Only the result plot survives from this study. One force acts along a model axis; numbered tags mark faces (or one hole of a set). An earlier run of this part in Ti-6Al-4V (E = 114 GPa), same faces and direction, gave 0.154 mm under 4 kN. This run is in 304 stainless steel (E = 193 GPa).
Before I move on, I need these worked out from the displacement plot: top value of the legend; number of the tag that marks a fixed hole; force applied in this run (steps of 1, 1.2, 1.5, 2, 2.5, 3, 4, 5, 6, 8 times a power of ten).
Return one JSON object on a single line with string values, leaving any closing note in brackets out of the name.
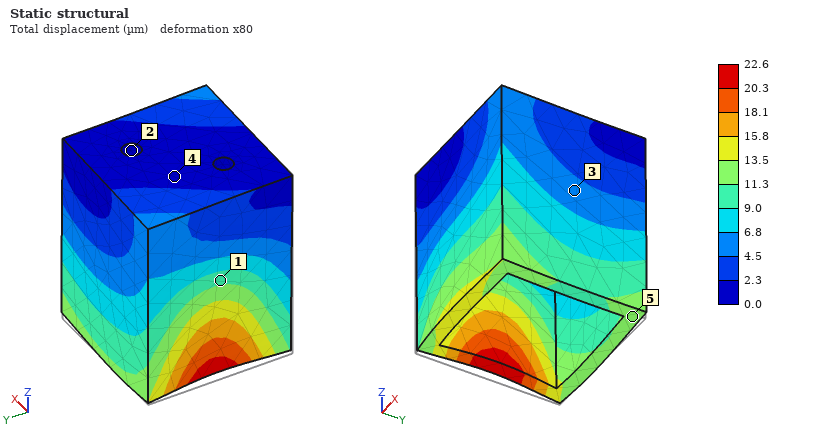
{"top value of the legend": "22.6 µm", "number of the tag that marks a fixed hole": "2", "force applied in this run": "1 kN"}
